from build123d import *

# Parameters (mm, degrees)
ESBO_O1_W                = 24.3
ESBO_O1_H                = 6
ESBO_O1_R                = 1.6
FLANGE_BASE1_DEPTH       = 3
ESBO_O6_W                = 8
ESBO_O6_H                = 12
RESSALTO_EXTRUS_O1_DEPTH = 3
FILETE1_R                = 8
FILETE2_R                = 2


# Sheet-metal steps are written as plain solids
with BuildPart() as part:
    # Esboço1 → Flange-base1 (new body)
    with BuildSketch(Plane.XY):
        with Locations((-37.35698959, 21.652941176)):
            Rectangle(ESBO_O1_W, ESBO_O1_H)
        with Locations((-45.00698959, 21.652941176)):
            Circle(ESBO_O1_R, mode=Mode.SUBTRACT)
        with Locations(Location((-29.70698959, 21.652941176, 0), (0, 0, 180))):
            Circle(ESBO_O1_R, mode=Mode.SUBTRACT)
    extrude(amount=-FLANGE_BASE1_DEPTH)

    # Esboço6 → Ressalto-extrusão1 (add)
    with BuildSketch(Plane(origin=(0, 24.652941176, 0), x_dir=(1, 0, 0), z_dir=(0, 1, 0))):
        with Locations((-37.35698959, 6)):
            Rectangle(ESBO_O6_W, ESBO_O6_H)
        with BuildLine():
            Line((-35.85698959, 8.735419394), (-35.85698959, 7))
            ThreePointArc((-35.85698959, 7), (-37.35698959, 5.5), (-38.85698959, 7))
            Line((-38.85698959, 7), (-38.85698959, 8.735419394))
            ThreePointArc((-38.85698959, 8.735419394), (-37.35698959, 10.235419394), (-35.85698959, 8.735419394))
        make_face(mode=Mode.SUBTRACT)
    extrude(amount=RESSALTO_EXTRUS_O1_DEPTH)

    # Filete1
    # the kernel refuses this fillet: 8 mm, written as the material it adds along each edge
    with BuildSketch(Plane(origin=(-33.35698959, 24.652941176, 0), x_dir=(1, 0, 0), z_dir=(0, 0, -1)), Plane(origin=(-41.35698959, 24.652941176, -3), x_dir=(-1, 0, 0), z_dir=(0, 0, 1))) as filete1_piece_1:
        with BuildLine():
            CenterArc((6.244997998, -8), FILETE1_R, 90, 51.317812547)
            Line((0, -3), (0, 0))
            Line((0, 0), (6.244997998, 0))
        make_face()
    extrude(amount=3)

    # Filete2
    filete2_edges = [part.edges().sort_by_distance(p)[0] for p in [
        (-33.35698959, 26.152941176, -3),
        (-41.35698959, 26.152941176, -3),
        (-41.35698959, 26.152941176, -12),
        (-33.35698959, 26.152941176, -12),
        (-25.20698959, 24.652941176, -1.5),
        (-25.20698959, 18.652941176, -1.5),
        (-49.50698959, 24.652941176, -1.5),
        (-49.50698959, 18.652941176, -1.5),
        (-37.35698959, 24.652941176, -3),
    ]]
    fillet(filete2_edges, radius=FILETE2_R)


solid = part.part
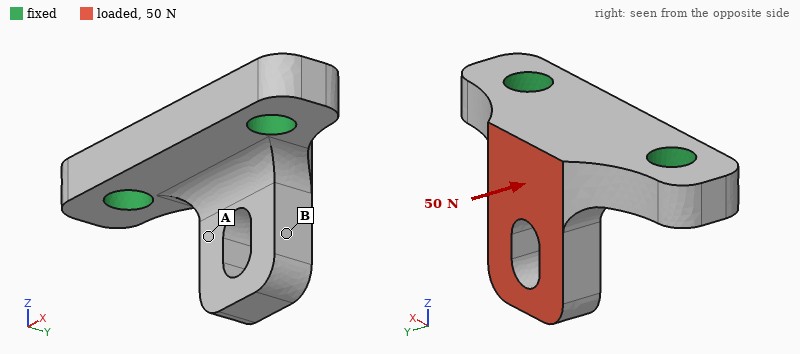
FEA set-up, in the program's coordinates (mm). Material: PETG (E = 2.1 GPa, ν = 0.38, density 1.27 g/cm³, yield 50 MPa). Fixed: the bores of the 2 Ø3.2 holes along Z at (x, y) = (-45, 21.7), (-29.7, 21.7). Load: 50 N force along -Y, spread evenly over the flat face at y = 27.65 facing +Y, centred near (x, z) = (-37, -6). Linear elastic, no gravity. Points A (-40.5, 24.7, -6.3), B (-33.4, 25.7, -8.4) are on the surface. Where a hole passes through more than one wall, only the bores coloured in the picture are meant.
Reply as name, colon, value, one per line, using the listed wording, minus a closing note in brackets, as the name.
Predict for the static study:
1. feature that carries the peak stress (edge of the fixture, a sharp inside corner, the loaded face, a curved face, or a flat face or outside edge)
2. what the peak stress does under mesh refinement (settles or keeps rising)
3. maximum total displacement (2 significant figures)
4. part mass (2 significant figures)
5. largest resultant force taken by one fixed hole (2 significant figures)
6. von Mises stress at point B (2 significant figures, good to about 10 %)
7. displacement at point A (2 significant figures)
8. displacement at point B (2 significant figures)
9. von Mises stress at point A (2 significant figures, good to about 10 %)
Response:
feature that carries the peak stress: edge of the fixture
what the peak stress does under mesh refinement: keeps rising
maximum total displacement: 0.27 mm
part mass: 0.85 g
largest resultant force taken by one fixed hole: 28 N
von Mises stress at point B: 2.5 MPa
displacement at point A: 0.092 mm
displacement at point B: 0.15 mm
von Mises stress at point A: 6.8 MPa
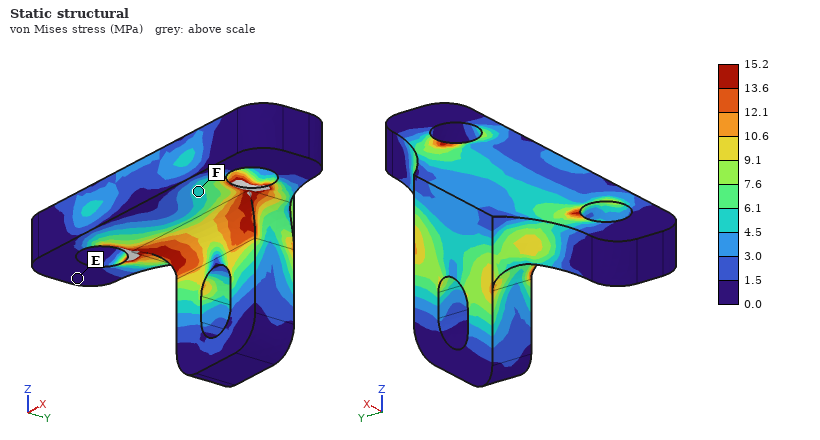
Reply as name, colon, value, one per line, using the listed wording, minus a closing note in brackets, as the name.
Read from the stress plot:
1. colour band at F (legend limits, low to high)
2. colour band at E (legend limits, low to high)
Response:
colour band at F: 4.5 to 6.1 MPa
colour band at E: 0.0 to 1.5 MPa
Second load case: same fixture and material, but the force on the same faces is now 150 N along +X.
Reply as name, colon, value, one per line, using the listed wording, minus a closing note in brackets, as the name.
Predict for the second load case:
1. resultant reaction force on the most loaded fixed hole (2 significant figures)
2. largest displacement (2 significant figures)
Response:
resultant reaction force on the most loaded fixed hole: 110 N
largest displacement: 0.21 mm
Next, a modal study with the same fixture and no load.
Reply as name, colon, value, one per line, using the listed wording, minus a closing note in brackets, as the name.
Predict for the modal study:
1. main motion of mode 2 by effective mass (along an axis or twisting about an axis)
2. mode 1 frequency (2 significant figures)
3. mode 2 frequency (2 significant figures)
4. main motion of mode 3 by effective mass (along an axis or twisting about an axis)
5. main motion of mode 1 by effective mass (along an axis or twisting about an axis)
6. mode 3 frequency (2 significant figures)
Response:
main motion of mode 2 by effective mass: along X
mode 1 frequency: 4600 Hz
mode 2 frequency: 8800 Hz
main motion of mode 3 by effective mass: along Z
main motion of mode 1 by effective mass: along Y
mode 3 frequency: 11 kHz
